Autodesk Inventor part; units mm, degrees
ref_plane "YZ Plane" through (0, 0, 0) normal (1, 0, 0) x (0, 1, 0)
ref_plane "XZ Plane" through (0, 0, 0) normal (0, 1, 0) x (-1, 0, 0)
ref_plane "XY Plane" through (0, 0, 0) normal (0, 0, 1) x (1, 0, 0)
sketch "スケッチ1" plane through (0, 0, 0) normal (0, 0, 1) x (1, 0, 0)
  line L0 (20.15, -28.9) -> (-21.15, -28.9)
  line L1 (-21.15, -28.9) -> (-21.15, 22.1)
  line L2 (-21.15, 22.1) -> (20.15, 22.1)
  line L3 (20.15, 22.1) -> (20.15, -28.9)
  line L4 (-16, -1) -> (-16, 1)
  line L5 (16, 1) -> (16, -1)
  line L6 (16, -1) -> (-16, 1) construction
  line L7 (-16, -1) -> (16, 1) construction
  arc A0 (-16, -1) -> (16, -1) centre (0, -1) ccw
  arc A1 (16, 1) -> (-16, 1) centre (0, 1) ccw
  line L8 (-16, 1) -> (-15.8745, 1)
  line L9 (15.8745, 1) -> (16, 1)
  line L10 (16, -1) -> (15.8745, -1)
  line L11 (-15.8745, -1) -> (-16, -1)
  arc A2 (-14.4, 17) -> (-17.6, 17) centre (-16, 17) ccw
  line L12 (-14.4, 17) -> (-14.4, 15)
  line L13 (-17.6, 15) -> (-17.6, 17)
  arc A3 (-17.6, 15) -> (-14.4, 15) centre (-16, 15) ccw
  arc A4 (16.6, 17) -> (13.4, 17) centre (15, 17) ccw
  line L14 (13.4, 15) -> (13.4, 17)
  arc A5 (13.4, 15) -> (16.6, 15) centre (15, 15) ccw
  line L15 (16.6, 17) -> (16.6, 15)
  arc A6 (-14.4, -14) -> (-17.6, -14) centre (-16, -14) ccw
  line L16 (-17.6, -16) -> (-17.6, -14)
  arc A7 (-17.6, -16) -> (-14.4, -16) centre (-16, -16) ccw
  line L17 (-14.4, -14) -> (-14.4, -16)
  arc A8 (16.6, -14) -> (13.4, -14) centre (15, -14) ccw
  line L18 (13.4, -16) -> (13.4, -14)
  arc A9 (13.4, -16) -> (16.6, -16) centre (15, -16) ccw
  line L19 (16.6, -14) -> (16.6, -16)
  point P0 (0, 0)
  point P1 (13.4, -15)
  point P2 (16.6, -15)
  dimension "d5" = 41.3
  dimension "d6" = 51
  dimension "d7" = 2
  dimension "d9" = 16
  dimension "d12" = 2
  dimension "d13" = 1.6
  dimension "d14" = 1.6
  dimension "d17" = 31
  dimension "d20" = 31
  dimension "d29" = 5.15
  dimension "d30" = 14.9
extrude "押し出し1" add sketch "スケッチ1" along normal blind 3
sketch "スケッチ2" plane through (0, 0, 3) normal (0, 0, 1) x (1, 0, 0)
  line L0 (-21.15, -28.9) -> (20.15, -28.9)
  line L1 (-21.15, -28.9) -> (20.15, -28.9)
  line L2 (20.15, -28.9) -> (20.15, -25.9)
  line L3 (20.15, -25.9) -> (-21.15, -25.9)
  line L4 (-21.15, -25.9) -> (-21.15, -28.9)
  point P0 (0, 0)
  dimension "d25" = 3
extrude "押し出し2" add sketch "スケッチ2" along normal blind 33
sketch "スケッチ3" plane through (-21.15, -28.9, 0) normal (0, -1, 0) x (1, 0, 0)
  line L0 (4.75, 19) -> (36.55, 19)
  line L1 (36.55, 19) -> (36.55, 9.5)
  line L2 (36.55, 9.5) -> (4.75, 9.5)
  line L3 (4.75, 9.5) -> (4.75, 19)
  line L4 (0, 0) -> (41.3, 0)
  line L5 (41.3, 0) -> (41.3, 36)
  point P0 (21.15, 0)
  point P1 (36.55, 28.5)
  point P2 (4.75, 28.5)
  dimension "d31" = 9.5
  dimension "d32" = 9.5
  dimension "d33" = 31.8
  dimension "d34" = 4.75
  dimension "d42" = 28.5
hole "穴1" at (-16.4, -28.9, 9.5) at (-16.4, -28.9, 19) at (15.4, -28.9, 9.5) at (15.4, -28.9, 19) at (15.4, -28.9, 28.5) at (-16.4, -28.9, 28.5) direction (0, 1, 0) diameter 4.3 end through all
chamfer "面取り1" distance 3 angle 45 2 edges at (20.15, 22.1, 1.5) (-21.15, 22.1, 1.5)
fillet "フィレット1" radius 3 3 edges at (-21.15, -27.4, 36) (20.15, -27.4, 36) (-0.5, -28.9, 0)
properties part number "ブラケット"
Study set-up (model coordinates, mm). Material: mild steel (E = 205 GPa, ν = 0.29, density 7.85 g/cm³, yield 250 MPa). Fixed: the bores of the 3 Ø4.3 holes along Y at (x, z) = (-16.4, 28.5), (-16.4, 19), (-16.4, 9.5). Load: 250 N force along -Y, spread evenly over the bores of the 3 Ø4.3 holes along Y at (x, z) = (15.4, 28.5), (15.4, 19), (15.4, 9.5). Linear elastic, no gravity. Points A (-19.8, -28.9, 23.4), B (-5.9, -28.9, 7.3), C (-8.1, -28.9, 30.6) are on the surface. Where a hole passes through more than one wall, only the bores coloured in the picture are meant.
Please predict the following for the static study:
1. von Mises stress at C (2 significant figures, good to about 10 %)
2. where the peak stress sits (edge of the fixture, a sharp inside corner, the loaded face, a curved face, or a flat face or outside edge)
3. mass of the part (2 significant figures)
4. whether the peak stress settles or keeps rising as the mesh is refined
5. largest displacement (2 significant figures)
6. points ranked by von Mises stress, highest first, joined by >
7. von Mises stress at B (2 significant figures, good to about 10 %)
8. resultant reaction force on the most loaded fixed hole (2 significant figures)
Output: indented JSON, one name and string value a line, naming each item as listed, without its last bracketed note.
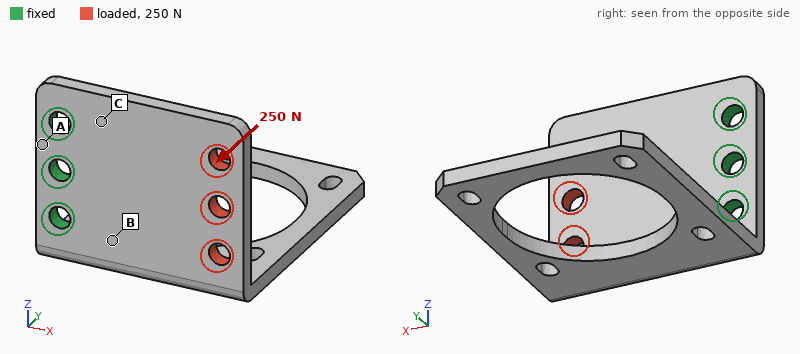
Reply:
{
  "von Mises stress at C": "67 MPa",
  "where the peak stress sits": "edge of the fixture",
  "mass of the part": "57 g",
  "whether the peak stress settles or keeps rising as the mesh is refined": "keeps rising",
  "largest displacement": "0.13 mm",
  "points ranked by von Mises stress, highest first, joined by >": "C > B > A",
  "von Mises stress at B": "33 MPa",
  "resultant reaction force on the most loaded fixed hole": "110 N"
}
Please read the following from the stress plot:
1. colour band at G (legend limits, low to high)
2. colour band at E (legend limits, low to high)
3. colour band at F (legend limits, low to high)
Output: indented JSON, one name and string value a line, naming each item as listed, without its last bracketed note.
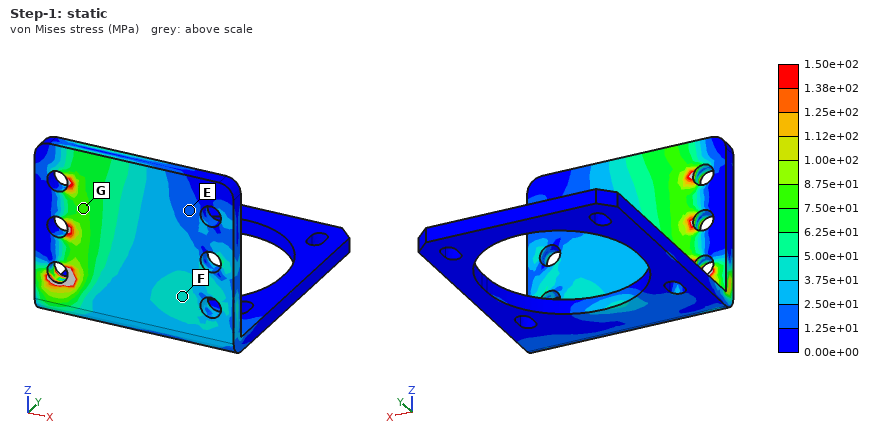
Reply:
{
  "colour band at G": "7.50e+01 to 8.75e+01 MPa",
  "colour band at E": "1.25e+01 to 2.50e+01 MPa",
  "colour band at F": "3.75e+01 to 5.00e+01 MPa"
}
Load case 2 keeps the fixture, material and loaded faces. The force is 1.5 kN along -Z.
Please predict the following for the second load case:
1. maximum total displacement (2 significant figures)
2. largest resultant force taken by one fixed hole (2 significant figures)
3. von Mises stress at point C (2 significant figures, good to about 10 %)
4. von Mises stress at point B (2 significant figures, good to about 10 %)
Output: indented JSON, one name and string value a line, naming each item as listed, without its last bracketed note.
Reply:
{
  "maximum total displacement": "22 µm",
  "largest resultant force taken by one fixed hole": "2.1 kN",
  "von Mises stress at point C": "45 MPa",
  "von Mises stress at point B": "41 MPa"
}
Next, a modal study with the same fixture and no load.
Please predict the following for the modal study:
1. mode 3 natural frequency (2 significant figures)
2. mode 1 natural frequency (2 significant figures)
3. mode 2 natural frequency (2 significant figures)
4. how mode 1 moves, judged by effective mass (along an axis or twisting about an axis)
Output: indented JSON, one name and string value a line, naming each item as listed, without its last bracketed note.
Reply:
{
  "mode 3 natural frequency": "2000 Hz",
  "mode 1 natural frequency": "750 Hz",
  "mode 2 natural frequency": "1300 Hz",
  "how mode 1 moves, judged by effective mass": "along Z"
}
